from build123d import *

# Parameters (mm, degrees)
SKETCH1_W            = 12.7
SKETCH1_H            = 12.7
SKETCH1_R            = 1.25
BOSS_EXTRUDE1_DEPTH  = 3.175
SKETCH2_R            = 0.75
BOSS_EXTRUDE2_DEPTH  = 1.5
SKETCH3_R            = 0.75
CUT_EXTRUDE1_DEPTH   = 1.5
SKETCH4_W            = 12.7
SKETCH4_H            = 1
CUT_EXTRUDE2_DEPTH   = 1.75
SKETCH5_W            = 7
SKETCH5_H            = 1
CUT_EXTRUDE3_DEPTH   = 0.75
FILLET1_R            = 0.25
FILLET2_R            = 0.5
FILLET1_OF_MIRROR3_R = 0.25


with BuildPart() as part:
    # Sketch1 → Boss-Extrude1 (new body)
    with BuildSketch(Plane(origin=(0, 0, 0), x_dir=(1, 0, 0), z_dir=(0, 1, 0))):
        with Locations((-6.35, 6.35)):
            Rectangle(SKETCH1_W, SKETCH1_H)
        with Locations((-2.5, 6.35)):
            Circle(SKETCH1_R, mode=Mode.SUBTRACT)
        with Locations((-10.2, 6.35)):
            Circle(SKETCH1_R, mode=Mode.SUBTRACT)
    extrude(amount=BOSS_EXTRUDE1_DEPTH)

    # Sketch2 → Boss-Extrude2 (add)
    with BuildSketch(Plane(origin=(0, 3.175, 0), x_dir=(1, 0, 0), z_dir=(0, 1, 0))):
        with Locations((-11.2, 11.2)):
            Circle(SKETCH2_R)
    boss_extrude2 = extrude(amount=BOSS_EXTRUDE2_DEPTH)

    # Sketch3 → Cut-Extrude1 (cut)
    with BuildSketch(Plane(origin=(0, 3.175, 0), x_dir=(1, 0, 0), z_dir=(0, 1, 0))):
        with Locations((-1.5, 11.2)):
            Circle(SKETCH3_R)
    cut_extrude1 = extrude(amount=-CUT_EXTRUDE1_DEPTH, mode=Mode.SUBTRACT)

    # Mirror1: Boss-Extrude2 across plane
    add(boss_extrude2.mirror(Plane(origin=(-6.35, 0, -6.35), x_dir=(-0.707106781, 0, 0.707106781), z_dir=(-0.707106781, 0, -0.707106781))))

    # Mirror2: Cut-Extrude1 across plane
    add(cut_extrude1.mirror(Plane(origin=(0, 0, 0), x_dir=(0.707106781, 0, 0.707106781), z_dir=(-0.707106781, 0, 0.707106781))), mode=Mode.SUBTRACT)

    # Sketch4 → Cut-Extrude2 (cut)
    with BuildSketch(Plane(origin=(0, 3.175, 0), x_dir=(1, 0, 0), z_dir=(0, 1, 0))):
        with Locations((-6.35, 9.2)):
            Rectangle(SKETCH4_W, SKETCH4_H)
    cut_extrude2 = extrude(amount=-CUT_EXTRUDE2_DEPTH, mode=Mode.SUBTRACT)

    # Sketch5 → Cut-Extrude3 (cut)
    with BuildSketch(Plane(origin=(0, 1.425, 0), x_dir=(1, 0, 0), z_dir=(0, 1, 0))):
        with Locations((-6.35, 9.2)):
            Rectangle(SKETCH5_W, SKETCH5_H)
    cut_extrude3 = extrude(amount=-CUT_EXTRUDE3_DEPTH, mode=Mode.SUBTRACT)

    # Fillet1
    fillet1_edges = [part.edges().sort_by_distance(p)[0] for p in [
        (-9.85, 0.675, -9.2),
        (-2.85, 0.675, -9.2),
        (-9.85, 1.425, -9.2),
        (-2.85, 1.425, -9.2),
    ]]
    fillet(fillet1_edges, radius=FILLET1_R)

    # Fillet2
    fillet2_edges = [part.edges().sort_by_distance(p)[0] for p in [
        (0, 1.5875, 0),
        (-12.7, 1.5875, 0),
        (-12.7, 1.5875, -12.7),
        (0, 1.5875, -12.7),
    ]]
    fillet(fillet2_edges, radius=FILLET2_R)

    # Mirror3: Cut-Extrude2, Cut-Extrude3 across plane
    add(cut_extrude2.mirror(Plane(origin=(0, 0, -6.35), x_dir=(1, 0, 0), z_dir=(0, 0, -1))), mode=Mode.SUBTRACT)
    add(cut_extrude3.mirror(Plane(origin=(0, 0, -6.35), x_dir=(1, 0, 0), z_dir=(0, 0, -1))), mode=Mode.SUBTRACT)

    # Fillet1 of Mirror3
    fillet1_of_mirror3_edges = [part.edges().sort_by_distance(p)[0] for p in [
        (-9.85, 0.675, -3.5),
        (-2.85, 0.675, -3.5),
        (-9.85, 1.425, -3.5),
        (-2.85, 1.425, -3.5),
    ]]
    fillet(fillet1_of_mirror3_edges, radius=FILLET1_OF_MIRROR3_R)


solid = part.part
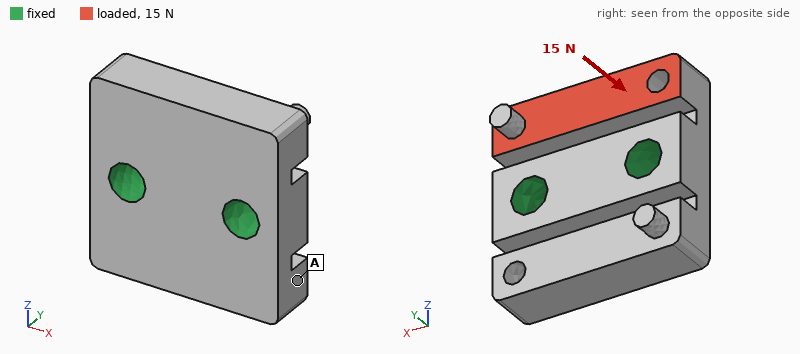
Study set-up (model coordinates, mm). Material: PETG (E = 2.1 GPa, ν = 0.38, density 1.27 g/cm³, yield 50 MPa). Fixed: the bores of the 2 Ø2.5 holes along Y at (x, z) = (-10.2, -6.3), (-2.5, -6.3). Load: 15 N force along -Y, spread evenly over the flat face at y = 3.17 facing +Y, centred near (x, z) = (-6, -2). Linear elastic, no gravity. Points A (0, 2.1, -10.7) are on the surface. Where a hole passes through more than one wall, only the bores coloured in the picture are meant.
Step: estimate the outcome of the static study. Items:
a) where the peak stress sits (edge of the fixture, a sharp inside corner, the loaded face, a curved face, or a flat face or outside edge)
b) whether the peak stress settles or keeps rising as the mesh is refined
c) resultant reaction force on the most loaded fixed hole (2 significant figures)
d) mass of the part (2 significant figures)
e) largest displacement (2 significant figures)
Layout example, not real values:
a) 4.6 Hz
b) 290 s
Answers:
a) a sharp inside corner
b) keeps rising
c) 7.5 N
d) 0.54 g
e) 90 µm
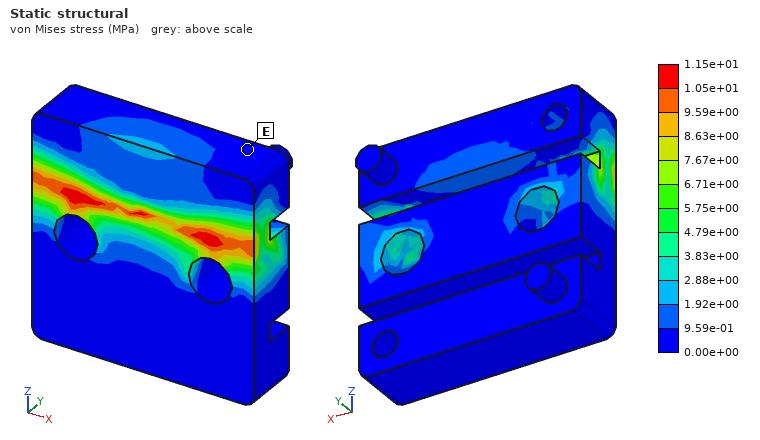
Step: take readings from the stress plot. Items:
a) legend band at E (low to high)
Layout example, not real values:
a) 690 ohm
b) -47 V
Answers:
a) 0.00e+00 to 9.59e-01 MPa
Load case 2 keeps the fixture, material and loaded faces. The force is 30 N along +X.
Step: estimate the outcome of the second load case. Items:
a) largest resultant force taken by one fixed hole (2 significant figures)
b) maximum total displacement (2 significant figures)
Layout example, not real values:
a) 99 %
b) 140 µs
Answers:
a) 20 N
b) 43 µm
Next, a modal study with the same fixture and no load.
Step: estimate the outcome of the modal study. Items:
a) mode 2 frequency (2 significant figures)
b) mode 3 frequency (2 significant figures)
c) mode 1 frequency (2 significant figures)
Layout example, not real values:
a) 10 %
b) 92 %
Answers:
a) 6200 Hz
b) 13 kHz
c) 6100 Hz
